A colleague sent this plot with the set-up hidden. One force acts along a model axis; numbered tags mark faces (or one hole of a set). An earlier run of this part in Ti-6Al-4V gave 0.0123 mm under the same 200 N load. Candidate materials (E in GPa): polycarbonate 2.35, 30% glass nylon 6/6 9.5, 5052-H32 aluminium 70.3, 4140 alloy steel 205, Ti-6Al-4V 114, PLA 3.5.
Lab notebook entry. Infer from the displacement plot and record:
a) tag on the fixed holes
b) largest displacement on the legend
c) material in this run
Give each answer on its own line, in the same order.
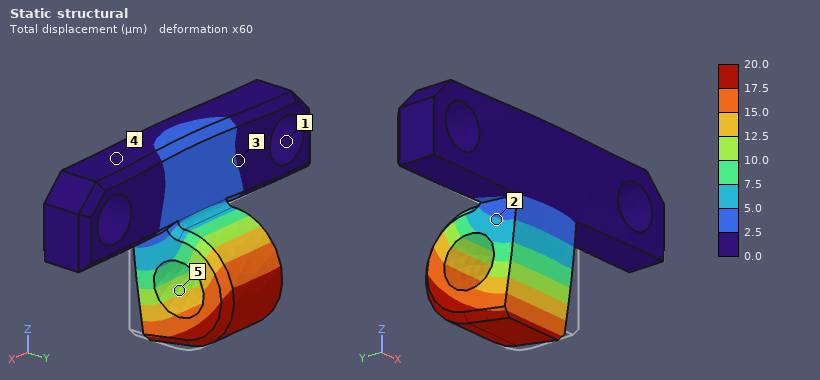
1
20.0 µm
5052-H32 aluminium
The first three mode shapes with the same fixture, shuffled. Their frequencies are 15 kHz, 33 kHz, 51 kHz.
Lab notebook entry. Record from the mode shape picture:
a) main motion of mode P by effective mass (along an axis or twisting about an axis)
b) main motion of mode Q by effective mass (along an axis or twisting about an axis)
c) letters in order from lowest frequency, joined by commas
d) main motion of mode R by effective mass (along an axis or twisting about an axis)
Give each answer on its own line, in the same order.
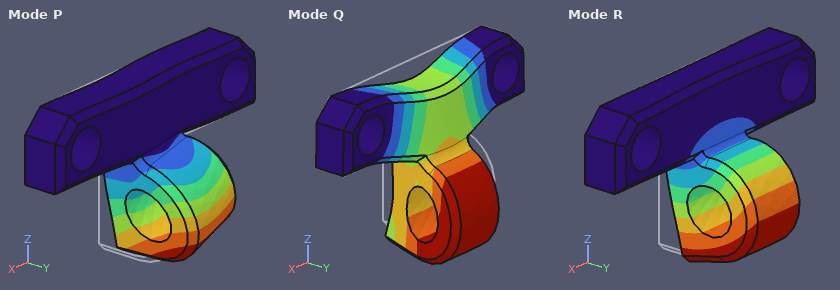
along X
along Z
R, P, Q
along Y
